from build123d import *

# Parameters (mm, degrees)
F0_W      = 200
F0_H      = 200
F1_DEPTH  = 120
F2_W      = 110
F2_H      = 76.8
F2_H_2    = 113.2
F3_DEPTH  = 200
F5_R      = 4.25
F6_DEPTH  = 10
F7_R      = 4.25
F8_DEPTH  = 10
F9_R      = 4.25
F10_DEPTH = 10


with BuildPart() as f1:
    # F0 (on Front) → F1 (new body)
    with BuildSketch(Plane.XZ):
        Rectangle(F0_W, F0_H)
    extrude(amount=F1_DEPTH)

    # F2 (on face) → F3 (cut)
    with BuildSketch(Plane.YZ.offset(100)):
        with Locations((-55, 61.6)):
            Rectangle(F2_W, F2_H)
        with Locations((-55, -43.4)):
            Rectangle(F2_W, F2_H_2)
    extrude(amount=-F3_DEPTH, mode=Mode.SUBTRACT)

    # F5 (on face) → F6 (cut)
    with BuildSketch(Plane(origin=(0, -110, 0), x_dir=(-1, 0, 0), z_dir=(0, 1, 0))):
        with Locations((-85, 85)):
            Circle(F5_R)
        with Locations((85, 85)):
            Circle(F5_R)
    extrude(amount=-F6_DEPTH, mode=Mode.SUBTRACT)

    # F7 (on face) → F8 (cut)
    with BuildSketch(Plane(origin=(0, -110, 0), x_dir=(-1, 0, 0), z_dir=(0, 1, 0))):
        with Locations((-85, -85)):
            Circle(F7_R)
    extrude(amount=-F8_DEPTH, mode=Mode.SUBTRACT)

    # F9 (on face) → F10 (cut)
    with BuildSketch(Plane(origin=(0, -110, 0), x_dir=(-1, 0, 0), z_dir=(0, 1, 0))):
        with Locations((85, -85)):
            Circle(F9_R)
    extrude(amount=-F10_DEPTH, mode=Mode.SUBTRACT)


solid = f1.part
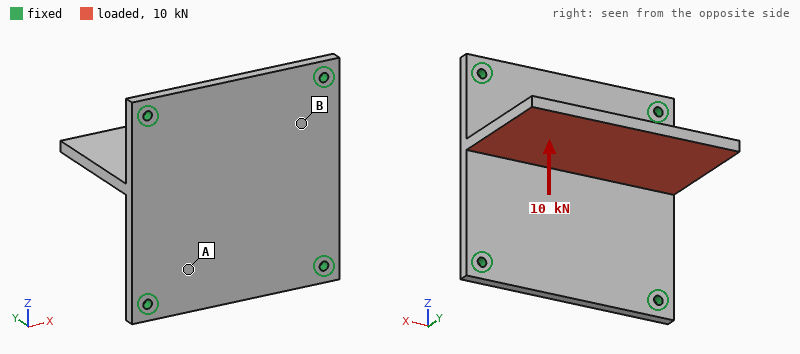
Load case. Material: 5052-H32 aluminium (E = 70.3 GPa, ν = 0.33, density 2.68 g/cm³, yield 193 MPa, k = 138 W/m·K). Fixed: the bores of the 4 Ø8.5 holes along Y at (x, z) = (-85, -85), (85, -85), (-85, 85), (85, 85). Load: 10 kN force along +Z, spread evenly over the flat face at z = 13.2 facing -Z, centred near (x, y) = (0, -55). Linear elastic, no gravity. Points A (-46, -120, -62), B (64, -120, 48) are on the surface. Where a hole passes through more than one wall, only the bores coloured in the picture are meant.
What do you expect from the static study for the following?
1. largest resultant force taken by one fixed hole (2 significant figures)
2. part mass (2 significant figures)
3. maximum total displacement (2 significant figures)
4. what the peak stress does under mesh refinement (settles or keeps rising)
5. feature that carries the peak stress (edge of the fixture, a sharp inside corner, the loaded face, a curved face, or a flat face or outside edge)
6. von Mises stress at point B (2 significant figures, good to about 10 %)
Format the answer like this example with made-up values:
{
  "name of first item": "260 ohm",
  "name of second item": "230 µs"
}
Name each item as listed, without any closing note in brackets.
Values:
{
  "largest resultant force taken by one fixed hole": "3.6 kN",
  "part mass": "1.7 kg",
  "maximum total displacement": "2.1 mm",
  "what the peak stress does under mesh refinement": "keeps rising",
  "feature that carries the peak stress": "edge of the fixture",
  "von Mises stress at point B": "34 MPa"
}
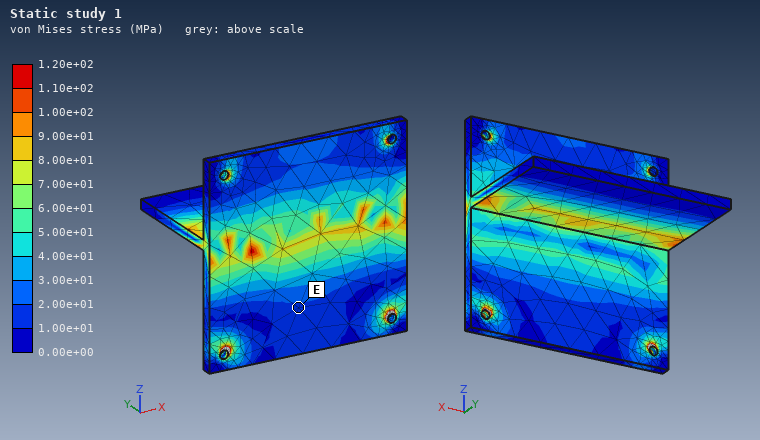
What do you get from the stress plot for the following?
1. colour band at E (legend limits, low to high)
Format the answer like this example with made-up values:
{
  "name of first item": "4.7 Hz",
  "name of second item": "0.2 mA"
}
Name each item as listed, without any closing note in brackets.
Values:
{
  "colour band at E": "1.00e+01 to 2.00e+01 MPa"
}
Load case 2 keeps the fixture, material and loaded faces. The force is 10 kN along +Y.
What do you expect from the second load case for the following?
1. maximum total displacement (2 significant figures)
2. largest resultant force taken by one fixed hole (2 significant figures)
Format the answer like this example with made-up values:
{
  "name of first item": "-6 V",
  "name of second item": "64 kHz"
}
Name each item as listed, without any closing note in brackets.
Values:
{
  "maximum total displacement": "0.53 mm",
  "largest resultant force taken by one fixed hole": "3.0 kN"
}
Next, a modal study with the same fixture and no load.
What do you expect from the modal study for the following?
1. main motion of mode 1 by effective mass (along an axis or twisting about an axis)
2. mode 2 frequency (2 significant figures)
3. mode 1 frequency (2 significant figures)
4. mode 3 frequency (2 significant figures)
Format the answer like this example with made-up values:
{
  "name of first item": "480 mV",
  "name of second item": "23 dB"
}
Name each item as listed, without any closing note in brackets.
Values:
{
  "main motion of mode 1 by effective mass": "along Z",
  "mode 2 frequency": "910 Hz",
  "mode 1 frequency": "550 Hz",
  "mode 3 frequency": "920 Hz"
}
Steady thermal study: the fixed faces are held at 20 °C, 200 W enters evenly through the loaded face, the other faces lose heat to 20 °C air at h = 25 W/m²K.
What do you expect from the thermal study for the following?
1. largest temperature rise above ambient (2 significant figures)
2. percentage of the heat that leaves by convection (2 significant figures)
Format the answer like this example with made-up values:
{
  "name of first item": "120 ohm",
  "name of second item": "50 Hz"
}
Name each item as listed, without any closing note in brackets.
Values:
{
  "largest temperature rise above ambient": "64 K",
  "percentage of the heat that leaves by convection": "36 %"
}
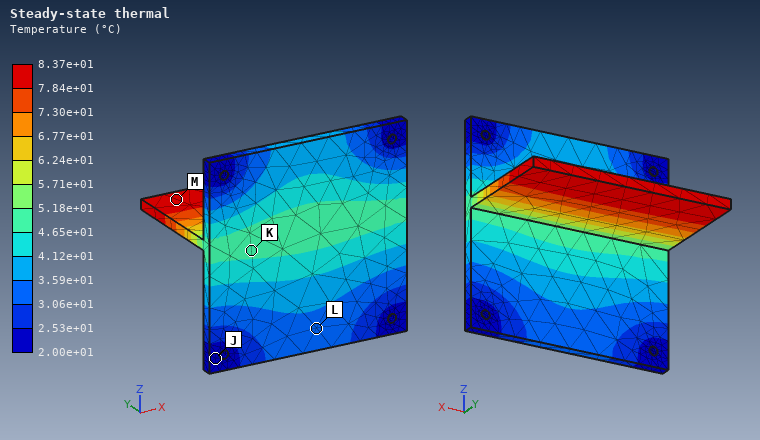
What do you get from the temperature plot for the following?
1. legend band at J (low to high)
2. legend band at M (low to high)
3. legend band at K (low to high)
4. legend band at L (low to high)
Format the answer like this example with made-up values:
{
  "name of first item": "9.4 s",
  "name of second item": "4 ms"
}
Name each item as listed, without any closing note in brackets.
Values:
{
  "legend band at J": "2.00e+01 to 2.53e+01 °C",
  "legend band at M": "7.84e+01 to 8.37e+01 °C",
  "legend band at K": "4.65e+01 to 5.18e+01 °C",
  "legend band at L": "3.06e+01 to 3.59e+01 °C"
}
